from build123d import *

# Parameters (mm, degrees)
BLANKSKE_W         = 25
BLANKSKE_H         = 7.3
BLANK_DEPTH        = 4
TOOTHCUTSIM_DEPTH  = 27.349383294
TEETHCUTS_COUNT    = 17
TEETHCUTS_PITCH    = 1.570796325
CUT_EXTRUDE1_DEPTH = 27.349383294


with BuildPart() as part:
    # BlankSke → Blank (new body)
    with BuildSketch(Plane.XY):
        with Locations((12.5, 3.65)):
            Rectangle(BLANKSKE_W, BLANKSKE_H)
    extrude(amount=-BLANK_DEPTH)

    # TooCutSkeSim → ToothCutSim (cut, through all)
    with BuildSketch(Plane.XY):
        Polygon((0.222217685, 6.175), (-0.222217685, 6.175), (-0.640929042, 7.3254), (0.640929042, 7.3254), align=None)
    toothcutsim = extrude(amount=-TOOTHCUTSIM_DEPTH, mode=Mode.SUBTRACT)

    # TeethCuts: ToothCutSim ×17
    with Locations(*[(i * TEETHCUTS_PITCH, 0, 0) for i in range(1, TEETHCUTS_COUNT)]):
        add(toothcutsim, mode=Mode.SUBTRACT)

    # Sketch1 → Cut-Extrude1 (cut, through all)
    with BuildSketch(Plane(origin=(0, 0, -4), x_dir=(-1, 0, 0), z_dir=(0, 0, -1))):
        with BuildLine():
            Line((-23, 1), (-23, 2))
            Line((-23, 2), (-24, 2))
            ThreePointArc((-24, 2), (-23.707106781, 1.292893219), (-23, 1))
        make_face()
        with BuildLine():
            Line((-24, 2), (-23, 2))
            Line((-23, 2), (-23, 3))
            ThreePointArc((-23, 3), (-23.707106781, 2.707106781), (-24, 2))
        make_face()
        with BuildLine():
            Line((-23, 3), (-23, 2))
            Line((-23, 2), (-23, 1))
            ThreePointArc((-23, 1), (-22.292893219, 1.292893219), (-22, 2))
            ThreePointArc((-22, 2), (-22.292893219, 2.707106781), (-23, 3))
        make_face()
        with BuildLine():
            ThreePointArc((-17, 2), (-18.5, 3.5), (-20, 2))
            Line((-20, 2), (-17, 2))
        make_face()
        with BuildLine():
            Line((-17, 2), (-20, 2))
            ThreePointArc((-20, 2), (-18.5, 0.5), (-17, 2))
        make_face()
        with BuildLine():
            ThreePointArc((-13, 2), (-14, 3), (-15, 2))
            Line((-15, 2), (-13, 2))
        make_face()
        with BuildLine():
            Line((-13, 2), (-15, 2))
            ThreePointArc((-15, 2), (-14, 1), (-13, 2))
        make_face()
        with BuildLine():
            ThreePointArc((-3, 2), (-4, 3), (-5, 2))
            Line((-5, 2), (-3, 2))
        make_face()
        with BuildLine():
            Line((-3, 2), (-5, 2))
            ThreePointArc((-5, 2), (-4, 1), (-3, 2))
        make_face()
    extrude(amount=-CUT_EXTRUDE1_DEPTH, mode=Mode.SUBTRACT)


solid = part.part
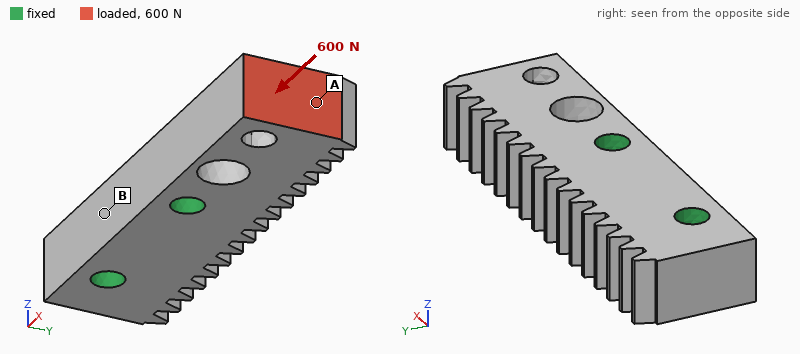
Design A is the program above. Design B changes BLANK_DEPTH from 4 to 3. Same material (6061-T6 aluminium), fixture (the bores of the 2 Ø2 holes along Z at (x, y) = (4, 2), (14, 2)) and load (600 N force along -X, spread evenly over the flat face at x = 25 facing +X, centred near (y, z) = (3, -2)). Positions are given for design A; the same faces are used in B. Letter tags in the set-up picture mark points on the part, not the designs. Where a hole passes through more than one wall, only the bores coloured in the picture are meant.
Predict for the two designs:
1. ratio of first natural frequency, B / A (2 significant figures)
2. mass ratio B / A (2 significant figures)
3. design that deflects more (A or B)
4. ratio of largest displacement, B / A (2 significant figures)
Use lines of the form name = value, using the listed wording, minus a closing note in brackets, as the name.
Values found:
ratio of first natural frequency, B / A = 0.80
mass ratio B / A = 0.75
design that deflects more = B
ratio of largest displacement, B / A = 1.3
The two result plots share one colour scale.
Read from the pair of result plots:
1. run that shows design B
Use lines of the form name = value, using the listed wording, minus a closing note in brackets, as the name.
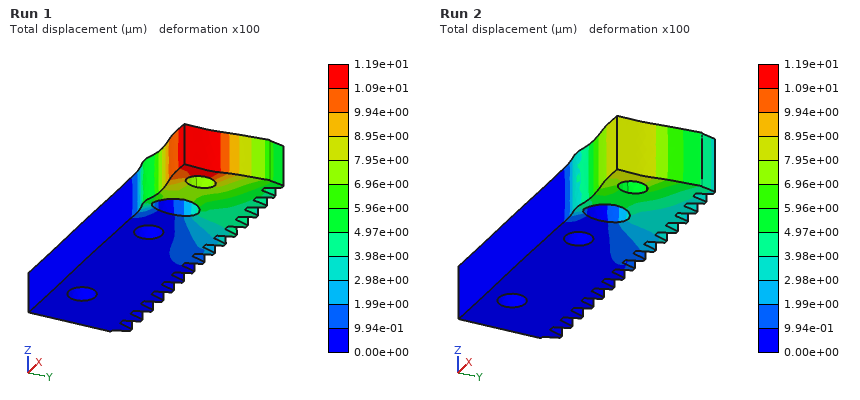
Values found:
run that shows design B = Run 1
